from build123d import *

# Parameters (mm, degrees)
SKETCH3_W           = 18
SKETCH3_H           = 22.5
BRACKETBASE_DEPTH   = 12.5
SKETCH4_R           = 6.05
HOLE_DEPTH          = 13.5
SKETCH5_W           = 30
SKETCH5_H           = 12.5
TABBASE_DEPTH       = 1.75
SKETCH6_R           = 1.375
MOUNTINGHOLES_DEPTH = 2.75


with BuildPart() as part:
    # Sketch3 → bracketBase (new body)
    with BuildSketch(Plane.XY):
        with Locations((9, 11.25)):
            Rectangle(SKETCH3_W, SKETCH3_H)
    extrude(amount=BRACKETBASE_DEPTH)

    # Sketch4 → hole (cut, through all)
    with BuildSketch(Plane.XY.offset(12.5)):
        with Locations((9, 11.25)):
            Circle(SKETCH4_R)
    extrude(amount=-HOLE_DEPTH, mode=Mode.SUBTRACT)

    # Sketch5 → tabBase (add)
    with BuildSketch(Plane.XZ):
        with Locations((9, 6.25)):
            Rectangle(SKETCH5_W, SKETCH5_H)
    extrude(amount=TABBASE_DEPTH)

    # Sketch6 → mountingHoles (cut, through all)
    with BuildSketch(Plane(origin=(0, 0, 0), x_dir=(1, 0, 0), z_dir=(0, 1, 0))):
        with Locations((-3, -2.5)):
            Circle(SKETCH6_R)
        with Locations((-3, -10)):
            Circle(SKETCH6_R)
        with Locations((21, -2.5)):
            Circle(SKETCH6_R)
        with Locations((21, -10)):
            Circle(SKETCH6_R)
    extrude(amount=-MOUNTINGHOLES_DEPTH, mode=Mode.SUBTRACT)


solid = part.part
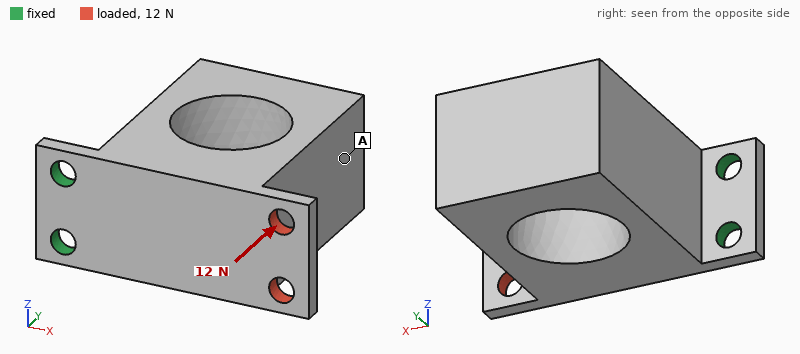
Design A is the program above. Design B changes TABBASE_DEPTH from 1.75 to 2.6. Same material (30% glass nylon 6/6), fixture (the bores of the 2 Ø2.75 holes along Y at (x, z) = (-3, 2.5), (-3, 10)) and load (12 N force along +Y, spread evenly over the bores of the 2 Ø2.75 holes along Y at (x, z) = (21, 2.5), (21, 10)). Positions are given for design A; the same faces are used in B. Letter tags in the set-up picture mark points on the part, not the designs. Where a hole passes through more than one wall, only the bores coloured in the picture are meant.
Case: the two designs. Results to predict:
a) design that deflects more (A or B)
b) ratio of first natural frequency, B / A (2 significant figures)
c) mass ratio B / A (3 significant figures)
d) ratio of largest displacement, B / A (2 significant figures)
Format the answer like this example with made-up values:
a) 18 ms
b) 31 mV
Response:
a) A
b) 1.6
c) 1.07
d) 0.37
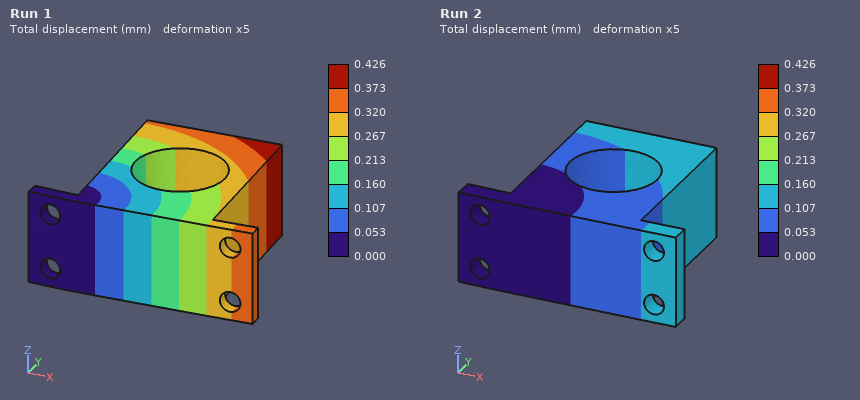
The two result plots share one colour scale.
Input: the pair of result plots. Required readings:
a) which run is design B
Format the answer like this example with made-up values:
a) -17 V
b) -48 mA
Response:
a) Run 2
